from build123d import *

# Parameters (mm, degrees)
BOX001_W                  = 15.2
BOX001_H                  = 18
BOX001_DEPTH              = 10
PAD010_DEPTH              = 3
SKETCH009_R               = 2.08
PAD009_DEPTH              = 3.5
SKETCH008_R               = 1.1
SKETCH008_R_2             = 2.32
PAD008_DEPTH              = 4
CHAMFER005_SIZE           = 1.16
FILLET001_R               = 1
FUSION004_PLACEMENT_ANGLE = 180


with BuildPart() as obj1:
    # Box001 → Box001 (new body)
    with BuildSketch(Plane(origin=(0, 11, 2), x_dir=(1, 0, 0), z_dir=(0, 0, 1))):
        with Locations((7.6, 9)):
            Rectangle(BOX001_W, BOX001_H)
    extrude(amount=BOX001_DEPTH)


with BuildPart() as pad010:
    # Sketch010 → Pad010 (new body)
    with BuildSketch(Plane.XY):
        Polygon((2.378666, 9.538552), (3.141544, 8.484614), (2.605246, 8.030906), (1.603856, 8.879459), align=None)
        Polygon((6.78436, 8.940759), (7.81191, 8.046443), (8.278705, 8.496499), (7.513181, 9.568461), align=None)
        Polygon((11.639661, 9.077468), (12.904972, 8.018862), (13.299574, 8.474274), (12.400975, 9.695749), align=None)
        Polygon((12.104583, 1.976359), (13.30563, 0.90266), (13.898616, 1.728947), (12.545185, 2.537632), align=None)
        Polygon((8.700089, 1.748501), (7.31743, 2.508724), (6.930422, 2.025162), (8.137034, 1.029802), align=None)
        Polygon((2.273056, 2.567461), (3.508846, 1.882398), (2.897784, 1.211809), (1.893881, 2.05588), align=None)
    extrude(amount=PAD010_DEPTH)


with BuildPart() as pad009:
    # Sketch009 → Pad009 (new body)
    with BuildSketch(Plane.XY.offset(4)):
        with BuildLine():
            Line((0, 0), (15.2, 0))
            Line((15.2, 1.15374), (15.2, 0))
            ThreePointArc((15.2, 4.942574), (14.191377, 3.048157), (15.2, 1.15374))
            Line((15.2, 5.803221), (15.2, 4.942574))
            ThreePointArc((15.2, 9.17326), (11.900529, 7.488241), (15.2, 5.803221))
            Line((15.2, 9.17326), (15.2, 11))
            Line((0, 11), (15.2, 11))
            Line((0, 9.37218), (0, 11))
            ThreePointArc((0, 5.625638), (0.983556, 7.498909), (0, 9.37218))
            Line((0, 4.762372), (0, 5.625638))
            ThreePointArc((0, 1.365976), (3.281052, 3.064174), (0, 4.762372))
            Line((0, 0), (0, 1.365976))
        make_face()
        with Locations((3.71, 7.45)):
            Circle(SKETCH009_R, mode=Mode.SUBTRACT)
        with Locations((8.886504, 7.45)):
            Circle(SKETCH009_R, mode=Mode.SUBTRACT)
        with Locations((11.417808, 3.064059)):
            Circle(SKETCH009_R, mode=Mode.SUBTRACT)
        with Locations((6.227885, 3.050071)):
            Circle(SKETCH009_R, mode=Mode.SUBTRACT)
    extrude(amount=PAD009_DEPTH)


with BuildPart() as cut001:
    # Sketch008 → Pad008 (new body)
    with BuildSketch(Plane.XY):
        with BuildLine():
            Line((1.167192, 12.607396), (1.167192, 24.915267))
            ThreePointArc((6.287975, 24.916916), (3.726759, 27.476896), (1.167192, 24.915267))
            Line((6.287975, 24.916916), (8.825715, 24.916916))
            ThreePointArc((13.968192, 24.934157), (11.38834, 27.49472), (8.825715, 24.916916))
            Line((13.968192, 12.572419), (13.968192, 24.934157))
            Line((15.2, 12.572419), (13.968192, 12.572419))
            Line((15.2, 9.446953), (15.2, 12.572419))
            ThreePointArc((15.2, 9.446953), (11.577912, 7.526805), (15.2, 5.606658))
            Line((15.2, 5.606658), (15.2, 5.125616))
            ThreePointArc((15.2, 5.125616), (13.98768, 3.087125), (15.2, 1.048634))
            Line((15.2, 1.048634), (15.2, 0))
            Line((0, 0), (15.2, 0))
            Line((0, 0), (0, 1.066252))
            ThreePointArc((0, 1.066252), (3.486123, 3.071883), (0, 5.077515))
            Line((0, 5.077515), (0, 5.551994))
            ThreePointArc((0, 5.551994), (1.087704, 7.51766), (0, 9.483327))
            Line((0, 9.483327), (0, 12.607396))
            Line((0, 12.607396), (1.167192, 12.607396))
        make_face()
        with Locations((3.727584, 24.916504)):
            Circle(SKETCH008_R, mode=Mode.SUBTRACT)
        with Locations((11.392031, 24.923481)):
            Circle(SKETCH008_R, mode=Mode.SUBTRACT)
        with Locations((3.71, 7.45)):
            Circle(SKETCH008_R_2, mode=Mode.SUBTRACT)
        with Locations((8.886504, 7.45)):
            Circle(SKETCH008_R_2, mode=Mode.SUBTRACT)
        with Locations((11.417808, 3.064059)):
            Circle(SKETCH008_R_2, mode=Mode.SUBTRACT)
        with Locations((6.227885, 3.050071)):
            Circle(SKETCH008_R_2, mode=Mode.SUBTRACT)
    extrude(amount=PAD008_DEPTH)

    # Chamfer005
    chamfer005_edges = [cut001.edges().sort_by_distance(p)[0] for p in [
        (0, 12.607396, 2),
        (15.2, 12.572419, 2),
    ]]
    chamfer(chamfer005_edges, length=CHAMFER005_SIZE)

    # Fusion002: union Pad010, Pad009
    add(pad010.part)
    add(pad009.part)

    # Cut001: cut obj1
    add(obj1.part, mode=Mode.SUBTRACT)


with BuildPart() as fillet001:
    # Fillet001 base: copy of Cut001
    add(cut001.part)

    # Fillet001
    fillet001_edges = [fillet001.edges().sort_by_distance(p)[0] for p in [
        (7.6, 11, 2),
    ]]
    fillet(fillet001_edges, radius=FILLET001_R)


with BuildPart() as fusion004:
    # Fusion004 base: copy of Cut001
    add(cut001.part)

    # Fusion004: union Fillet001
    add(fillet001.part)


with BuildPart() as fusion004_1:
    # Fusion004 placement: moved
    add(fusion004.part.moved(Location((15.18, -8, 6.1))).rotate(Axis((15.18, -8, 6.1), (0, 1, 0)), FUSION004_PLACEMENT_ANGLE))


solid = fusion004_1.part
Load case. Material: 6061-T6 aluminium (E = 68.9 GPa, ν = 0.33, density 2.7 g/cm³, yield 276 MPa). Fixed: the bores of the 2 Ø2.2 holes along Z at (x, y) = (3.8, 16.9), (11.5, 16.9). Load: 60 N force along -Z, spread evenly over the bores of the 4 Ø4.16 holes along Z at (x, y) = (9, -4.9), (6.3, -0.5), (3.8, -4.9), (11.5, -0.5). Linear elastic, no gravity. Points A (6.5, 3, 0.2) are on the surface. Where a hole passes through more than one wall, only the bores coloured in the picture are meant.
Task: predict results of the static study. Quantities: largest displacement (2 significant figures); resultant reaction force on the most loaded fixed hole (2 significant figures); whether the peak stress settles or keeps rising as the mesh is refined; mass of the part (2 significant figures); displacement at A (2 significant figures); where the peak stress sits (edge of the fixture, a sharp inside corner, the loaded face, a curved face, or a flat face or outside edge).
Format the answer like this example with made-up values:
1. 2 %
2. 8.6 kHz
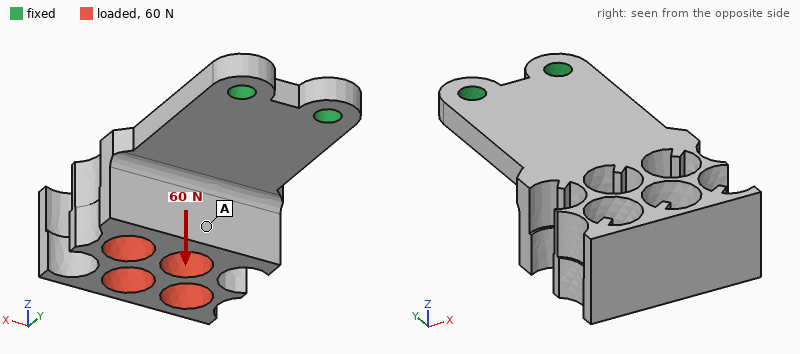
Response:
1. 0.35 mm
2. 30 N
3. keeps rising
4. 2.6 g
5. 0.16 mm
6. edge of the fixture
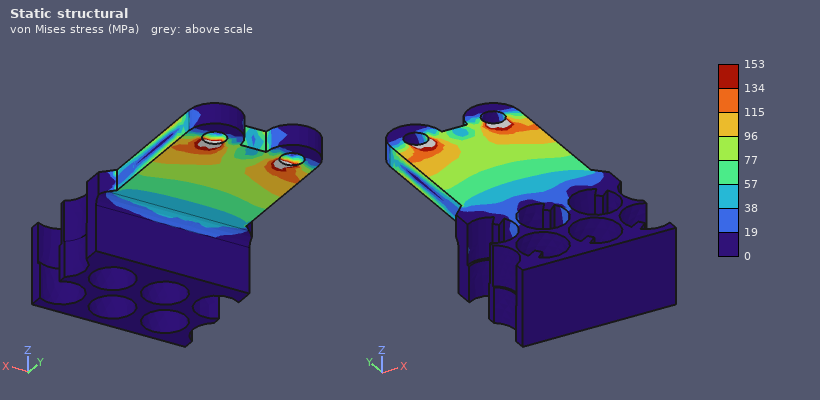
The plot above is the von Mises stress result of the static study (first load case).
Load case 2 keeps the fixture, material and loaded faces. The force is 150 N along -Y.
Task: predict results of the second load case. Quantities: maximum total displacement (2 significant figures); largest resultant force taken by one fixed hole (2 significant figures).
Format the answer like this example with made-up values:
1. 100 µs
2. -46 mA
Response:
1. 0.31 mm
2. 77 N
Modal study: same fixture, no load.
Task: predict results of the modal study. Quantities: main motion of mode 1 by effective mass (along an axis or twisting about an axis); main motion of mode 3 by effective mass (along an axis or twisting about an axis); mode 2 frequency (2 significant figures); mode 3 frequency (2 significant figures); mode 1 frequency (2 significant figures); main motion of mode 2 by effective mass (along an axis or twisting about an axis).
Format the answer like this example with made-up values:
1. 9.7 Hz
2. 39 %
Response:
1. along Z
2. along X
3. 6200 Hz
4. 9700 Hz
5. 1900 Hz
6. along X
